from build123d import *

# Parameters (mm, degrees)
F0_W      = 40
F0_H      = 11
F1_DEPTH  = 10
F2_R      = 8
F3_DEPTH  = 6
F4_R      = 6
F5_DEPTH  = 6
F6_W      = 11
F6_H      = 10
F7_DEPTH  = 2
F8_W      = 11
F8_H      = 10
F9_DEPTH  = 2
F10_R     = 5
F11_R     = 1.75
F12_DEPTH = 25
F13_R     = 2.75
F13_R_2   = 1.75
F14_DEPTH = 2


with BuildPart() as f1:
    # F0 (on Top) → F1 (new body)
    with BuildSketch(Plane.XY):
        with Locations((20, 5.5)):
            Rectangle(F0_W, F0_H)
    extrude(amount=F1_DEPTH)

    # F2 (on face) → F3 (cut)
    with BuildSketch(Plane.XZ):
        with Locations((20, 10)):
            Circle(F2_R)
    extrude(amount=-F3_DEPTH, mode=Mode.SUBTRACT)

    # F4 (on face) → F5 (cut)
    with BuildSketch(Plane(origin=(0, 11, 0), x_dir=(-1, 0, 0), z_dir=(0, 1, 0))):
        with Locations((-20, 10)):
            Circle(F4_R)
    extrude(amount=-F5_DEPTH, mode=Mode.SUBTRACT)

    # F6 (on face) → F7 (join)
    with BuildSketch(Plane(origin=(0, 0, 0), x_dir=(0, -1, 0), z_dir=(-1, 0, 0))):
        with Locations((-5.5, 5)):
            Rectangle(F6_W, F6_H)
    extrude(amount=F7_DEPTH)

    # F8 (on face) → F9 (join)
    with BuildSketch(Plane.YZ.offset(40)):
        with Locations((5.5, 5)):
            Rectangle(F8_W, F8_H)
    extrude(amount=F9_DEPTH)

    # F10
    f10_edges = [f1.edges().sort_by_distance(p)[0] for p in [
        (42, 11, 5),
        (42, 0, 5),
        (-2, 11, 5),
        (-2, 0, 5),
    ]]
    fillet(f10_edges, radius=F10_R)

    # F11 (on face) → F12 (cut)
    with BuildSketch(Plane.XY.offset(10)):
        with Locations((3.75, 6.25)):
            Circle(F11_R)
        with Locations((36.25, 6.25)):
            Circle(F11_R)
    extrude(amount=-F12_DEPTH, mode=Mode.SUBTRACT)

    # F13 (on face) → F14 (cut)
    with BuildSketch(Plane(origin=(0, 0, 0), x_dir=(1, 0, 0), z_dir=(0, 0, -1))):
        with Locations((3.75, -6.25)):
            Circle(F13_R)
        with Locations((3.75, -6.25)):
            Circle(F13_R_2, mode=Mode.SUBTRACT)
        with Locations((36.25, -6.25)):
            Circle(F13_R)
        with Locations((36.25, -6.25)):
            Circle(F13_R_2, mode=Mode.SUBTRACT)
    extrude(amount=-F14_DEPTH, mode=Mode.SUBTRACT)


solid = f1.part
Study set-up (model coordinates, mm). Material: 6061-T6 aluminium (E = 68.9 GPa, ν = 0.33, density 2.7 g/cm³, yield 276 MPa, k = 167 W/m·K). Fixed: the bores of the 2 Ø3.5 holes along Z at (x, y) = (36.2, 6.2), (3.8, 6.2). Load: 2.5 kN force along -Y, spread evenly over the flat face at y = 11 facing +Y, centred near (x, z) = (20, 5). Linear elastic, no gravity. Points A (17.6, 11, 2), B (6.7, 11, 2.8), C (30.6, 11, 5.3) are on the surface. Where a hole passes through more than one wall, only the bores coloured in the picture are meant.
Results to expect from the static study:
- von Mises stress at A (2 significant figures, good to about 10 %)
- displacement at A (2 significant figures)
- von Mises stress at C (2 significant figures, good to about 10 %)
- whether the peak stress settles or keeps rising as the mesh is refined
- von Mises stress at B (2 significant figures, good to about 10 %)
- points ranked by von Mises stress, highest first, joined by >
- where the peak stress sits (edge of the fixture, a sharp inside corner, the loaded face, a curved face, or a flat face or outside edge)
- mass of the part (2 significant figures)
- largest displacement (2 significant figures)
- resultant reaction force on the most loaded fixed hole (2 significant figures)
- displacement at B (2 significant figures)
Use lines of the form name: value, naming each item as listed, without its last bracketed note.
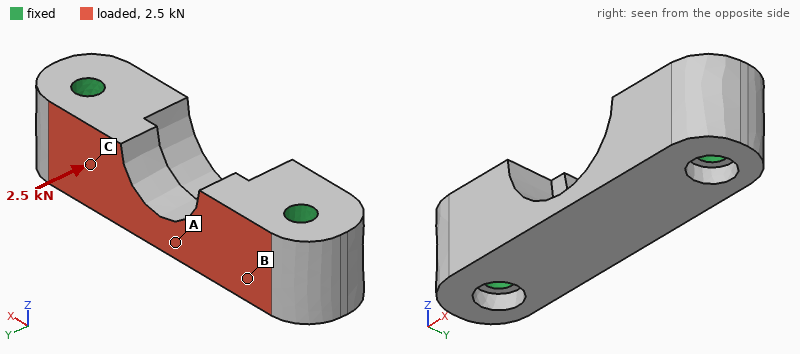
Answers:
von Mises stress at A: 36 MPa
displacement at A: 13 µm
von Mises stress at C: 11 MPa
whether the peak stress settles or keeps rising as the mesh is refined: keeps rising
von Mises stress at B: 19 MPa
points ranked by von Mises stress, highest first, joined by >: A > B > C
where the peak stress sits: edge of the fixture
mass of the part: 9.4 g
largest displacement: 15 µm
resultant reaction force on the most loaded fixed hole: 1.3 kN
displacement at B: 5.0 µm
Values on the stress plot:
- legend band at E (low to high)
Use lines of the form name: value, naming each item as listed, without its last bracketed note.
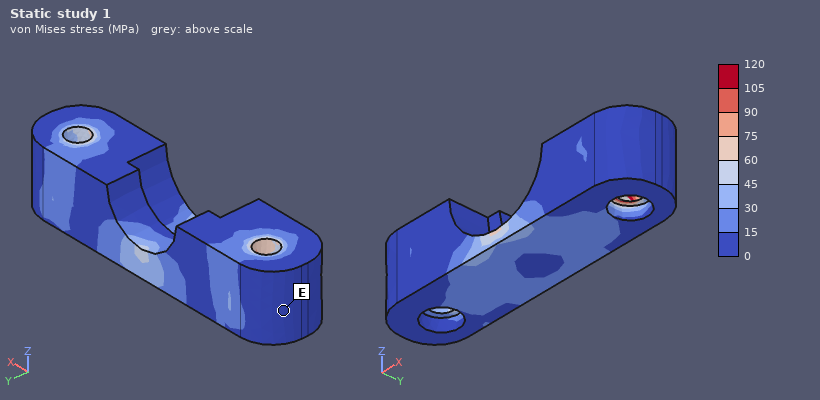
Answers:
legend band at E: 0 to 15 MPa
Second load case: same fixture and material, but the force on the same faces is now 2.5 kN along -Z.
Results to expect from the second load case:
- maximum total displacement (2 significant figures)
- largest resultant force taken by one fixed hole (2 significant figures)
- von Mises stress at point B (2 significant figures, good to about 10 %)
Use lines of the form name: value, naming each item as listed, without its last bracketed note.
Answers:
maximum total displacement: 20 µm
largest resultant force taken by one fixed hole: 1.3 kN
von Mises stress at point B: 39 MPa
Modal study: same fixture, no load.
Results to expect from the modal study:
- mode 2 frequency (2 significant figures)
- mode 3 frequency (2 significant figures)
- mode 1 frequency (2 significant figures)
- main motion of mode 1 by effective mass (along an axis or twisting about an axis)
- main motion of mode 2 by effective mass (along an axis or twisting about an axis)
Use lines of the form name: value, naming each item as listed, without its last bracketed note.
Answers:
mode 2 frequency: 37 kHz
mode 3 frequency: 51 kHz
mode 1 frequency: 30 kHz
main motion of mode 1 by effective mass: along Y
main motion of mode 2 by effective mass: along Z
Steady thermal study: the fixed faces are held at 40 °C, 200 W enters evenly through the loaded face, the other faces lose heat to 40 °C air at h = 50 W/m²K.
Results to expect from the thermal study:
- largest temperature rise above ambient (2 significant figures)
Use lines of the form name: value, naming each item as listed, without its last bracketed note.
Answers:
largest temperature rise above ambient: 60 K
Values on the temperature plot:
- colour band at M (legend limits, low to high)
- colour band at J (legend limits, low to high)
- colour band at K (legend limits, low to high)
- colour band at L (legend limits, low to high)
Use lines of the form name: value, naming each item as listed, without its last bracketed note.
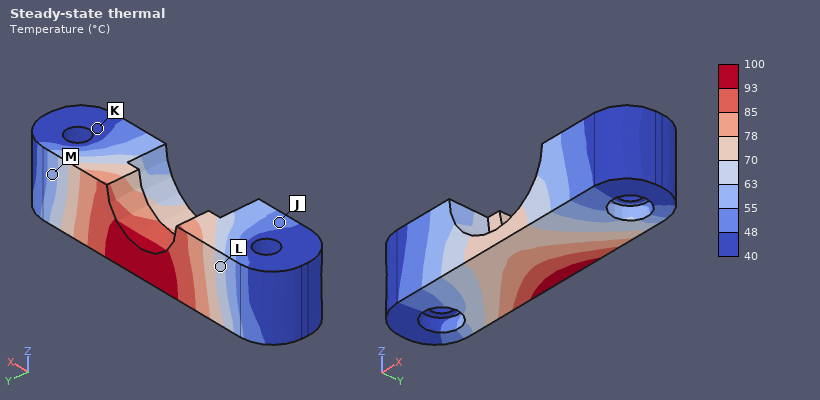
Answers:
colour band at M: 55 to 63 °C
colour band at J: 48 to 55 °C
colour band at K: 40 to 48 °C
colour band at L: 63 to 70 °C
